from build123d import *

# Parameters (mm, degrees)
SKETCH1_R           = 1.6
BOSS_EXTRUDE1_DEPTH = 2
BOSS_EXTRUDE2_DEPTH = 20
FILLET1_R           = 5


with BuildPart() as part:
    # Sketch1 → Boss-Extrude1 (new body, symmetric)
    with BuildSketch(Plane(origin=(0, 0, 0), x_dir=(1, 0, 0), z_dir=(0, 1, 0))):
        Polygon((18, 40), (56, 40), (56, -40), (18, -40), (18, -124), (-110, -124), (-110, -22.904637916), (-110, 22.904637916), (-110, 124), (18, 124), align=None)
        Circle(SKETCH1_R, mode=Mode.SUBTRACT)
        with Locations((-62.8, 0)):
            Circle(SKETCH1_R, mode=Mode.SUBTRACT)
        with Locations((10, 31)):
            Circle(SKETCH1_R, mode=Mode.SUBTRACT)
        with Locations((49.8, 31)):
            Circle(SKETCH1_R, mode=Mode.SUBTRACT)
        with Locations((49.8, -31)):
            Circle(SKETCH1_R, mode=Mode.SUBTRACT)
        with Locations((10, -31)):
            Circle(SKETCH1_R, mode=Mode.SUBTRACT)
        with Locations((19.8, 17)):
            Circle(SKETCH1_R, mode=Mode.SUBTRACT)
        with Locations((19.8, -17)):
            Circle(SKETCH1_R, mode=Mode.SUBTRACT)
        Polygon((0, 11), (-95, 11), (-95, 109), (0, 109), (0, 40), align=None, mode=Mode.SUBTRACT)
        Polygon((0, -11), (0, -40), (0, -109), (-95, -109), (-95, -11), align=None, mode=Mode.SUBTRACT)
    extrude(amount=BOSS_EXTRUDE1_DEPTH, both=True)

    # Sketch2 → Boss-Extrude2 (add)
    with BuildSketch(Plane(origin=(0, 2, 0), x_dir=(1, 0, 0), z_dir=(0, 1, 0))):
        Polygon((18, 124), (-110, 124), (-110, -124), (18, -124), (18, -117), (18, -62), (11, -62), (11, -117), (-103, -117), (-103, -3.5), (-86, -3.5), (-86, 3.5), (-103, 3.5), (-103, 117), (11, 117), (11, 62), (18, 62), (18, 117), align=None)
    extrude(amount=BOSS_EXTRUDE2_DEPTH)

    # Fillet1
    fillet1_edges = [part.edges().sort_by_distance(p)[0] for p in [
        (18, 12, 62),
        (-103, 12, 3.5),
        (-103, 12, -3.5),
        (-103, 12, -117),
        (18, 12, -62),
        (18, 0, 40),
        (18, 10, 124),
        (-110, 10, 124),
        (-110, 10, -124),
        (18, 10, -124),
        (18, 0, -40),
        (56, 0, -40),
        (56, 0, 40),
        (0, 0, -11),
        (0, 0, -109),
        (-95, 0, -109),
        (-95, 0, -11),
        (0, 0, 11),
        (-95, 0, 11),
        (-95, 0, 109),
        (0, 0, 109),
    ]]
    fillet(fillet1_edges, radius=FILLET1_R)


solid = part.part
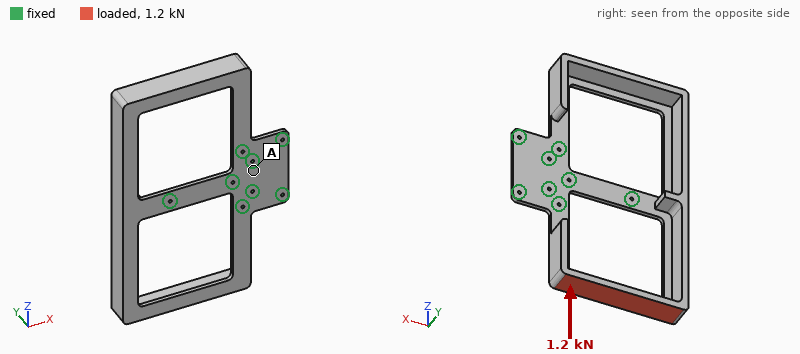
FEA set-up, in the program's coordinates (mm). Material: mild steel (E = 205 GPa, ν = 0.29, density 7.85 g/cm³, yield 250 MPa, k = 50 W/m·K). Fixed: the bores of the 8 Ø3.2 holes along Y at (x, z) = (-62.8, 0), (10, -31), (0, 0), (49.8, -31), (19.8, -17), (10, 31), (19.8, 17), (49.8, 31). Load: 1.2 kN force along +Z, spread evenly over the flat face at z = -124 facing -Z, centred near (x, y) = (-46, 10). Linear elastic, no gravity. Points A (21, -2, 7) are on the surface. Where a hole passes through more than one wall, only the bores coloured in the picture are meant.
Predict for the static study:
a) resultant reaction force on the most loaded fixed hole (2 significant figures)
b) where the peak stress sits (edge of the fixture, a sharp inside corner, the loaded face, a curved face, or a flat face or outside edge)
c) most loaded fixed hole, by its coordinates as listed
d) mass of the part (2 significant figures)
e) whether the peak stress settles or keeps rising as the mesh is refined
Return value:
860 N
edge of the fixture
(-62.8, 0)
1.2 kg
keeps rising
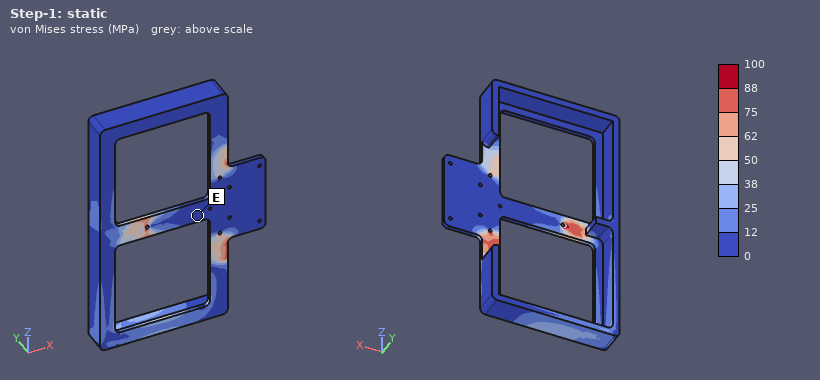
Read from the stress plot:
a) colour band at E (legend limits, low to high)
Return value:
0 to 12 MPa
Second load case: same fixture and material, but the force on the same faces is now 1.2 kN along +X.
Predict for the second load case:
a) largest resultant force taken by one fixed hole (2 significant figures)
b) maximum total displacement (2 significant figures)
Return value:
980 N
0.38 mm
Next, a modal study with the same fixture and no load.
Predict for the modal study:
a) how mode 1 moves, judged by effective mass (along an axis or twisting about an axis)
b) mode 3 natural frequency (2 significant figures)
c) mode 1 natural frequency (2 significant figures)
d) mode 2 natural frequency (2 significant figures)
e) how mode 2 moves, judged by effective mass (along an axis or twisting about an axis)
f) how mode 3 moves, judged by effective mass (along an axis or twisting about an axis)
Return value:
twisting about X
340 Hz
120 Hz
310 Hz
along Y
along Y
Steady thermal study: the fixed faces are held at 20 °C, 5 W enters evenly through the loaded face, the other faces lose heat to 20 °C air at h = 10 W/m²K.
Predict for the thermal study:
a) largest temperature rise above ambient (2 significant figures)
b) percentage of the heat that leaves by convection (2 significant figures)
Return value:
23 K
68 %
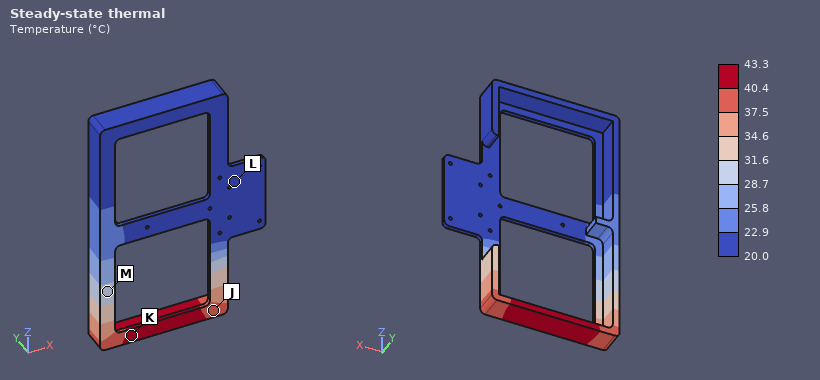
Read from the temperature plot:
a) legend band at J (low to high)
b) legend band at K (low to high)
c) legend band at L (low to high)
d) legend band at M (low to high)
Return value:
37.5 to 40.4 °C
40.4 to 43.3 °C
20.0 to 22.9 °C
28.7 to 31.6 °C
